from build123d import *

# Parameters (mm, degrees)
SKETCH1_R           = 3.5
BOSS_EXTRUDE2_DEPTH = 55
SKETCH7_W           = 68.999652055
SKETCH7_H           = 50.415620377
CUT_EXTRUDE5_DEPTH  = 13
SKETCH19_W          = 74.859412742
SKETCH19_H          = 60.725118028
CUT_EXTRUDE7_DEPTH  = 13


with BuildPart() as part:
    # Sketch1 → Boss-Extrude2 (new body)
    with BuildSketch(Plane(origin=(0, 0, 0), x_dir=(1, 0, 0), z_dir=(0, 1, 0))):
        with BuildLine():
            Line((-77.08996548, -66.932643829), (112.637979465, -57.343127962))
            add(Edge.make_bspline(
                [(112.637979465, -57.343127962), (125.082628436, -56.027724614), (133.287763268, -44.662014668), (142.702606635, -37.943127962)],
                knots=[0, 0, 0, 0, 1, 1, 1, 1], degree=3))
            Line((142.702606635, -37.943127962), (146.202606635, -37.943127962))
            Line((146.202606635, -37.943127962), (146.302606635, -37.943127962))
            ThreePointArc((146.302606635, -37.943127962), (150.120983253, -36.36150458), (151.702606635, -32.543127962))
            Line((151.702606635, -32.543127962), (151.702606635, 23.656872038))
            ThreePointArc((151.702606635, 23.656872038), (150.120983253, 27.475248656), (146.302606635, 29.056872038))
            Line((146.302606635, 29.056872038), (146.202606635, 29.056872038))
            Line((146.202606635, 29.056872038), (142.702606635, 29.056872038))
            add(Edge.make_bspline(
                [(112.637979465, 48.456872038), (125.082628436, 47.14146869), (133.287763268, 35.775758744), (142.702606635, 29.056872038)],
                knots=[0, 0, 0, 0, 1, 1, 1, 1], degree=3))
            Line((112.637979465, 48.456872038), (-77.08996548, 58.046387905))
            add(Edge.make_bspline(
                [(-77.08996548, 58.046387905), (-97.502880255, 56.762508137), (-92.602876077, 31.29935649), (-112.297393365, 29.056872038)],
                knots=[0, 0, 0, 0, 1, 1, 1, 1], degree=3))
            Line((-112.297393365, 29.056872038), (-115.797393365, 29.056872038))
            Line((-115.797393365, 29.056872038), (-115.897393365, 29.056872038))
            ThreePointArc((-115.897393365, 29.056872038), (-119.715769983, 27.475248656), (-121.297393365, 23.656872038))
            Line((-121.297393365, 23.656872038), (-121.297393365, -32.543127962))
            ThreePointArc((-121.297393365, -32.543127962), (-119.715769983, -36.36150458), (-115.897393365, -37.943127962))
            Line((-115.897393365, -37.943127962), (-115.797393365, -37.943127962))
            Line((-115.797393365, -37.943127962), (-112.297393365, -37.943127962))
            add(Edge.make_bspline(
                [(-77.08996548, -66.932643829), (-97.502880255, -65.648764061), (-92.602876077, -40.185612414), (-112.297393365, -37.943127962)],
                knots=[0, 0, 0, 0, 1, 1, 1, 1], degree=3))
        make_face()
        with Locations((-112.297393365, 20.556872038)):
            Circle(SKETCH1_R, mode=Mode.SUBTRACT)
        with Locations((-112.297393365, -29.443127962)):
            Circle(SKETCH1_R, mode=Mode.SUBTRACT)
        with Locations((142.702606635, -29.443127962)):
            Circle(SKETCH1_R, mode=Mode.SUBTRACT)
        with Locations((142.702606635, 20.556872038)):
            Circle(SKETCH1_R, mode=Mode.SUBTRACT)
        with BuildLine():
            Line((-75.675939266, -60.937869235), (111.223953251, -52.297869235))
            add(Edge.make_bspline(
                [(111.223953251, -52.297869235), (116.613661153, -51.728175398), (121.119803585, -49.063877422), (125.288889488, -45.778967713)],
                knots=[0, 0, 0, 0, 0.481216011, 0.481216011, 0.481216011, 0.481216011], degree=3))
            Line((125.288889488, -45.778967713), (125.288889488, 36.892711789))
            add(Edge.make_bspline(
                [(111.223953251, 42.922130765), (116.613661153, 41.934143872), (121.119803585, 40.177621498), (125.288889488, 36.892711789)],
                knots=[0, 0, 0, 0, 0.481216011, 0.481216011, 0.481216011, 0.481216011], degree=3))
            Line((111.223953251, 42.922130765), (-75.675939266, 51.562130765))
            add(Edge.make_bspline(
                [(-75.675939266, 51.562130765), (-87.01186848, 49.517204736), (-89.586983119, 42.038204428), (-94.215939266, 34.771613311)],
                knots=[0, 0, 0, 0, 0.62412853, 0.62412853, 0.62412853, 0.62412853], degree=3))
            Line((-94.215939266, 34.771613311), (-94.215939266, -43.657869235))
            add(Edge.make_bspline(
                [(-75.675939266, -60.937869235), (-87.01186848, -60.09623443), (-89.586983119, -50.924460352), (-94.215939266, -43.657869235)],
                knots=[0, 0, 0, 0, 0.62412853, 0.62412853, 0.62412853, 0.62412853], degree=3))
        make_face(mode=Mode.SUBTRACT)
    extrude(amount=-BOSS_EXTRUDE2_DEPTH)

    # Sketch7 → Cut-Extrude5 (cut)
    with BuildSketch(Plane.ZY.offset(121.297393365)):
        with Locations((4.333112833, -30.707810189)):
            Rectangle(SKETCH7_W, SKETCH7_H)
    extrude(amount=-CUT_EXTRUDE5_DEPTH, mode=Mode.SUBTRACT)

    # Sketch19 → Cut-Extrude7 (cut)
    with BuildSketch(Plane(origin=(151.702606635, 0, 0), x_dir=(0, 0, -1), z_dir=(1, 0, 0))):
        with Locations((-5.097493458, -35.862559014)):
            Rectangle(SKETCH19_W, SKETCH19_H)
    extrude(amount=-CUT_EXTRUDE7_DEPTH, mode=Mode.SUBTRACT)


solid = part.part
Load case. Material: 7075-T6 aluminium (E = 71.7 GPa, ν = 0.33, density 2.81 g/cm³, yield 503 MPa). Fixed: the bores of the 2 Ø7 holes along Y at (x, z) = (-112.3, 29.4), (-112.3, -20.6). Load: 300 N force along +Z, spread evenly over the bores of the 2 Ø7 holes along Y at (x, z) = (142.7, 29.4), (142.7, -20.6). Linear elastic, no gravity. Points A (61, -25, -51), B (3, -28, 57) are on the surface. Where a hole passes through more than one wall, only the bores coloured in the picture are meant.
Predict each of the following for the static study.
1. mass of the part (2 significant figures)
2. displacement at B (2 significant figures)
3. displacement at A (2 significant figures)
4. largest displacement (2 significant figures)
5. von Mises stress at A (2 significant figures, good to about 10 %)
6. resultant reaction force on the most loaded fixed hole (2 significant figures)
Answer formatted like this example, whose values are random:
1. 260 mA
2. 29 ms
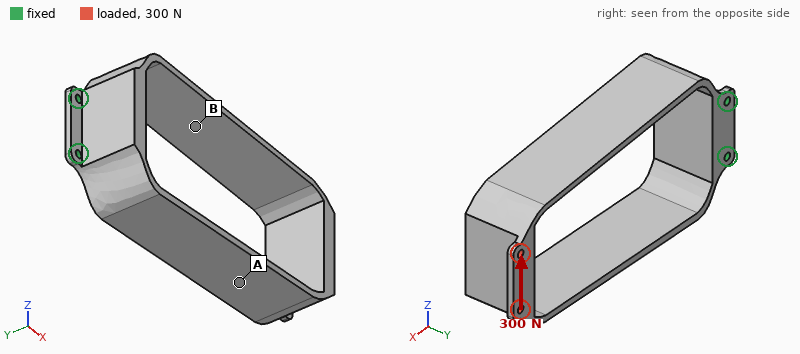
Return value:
1. 780 g
2. 1.3 mm
3. 2.2 mm
4. 2.8 mm
5. 21 MPa
6. 1.4 kN
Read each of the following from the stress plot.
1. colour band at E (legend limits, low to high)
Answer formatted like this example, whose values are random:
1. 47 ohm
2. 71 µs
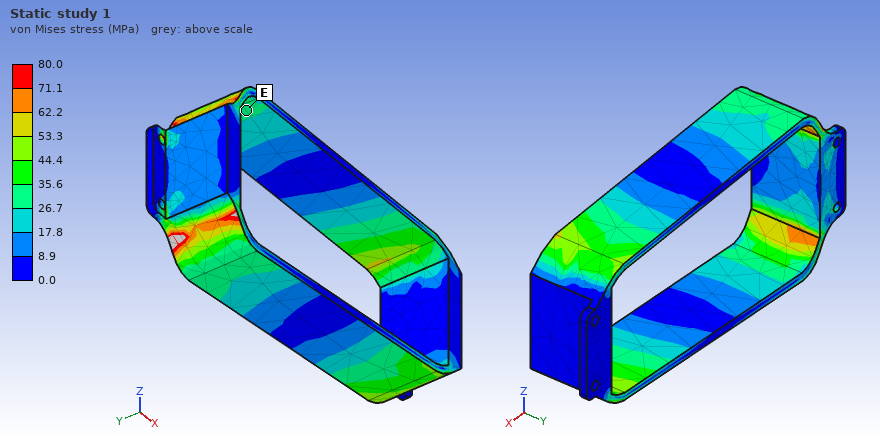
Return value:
1. 26.7 to 35.6 MPa
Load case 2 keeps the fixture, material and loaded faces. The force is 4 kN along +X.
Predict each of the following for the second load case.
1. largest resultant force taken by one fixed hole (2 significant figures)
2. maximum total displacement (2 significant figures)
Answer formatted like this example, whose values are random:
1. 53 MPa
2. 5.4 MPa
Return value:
1. 3.0 kN
2. 1.6 mm
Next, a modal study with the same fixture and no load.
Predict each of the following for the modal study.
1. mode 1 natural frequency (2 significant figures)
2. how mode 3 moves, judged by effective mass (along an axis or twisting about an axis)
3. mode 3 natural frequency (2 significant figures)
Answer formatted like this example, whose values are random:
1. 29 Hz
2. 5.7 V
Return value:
1. 91 Hz
2. twisting about X
3. 450 Hz
